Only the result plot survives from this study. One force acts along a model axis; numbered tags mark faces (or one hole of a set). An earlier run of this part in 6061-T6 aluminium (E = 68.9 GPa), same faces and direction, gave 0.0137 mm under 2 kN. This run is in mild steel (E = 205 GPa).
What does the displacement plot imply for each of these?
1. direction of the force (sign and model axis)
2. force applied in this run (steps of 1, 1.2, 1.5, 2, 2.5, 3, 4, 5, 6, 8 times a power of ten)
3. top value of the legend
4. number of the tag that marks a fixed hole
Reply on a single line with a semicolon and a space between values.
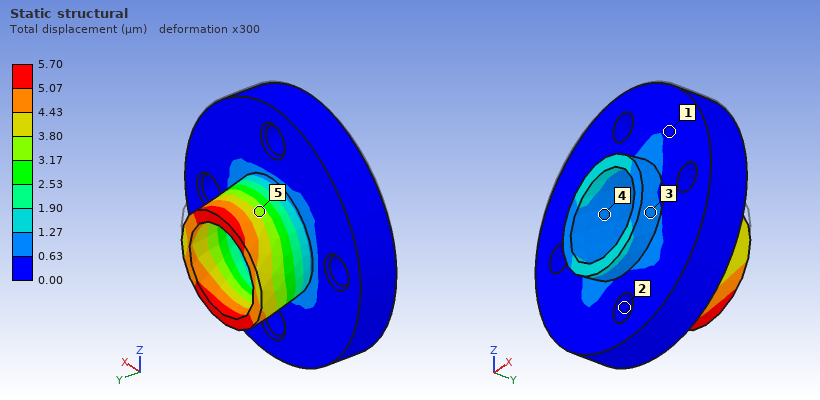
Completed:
-Z; 2.5 kN; 5.70 µm; 2
